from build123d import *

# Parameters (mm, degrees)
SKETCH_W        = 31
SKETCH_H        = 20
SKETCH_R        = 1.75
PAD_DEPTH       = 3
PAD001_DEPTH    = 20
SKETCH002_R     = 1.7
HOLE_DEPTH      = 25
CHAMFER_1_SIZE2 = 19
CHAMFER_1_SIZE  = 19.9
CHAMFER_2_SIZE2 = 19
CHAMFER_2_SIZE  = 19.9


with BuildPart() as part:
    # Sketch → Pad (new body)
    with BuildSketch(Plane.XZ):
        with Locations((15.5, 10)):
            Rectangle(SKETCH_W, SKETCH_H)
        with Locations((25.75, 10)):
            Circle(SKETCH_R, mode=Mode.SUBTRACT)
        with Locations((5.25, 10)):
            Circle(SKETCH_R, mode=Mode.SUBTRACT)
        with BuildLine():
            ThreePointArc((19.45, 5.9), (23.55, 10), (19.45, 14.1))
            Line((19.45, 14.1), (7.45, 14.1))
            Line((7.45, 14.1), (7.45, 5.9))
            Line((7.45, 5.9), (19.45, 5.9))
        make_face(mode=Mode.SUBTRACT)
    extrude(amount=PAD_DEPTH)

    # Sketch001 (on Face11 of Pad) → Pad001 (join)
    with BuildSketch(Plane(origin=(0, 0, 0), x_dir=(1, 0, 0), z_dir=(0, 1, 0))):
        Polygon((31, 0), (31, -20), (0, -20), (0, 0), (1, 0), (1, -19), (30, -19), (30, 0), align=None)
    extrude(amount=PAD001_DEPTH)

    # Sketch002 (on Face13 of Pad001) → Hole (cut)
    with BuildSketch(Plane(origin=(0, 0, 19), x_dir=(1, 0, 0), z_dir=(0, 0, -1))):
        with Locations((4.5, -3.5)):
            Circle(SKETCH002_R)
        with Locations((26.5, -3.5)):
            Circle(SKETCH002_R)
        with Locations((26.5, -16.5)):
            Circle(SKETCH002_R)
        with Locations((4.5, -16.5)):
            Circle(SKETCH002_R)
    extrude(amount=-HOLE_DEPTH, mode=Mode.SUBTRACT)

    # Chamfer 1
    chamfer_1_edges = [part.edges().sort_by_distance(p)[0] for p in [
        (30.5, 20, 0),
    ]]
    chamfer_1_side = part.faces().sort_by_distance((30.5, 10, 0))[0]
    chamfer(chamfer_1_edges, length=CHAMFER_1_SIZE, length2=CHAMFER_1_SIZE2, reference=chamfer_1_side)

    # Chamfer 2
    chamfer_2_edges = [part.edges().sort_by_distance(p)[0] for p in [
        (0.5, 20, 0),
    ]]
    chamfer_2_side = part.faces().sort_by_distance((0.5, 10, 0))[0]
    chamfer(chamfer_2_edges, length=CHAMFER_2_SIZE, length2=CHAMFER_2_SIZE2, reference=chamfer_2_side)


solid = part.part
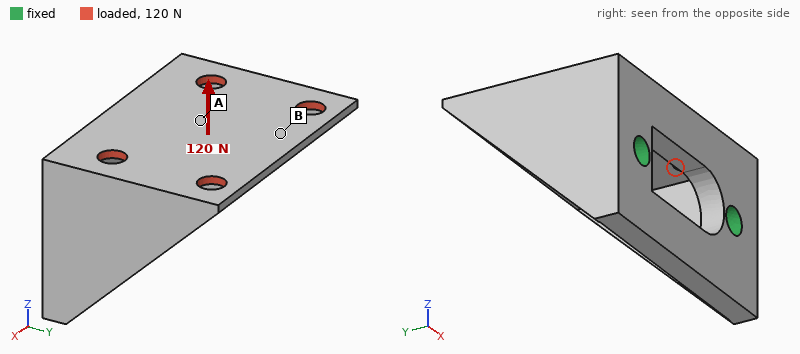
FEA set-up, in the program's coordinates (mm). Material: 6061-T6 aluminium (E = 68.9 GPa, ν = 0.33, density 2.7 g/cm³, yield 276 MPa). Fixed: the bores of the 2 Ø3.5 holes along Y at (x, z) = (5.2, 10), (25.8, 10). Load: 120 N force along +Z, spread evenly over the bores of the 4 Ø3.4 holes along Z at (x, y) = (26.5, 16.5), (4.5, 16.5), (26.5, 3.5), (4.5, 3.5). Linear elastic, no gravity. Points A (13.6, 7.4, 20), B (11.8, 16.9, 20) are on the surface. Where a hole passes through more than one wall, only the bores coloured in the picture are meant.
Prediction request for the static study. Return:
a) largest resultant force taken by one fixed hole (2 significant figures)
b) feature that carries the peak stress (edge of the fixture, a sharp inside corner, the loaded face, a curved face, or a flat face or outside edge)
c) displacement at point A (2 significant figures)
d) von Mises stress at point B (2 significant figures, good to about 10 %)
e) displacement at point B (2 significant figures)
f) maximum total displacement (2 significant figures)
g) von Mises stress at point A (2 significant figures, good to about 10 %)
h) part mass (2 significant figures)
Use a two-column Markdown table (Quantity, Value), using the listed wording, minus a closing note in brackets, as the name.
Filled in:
| Quantity | Value |
|---|---|
| largest resultant force taken by one fixed hole | 65 N |
| feature that carries the peak stress | the loaded face |
| displacement at point A | 0.033 mm |
| von Mises stress at point B | 17 MPa |
| displacement at point B | 0.085 mm |
| maximum total displacement | 0.11 mm |
| von Mises stress at point A | 8.1 MPa |
| part mass | 6.5 g |
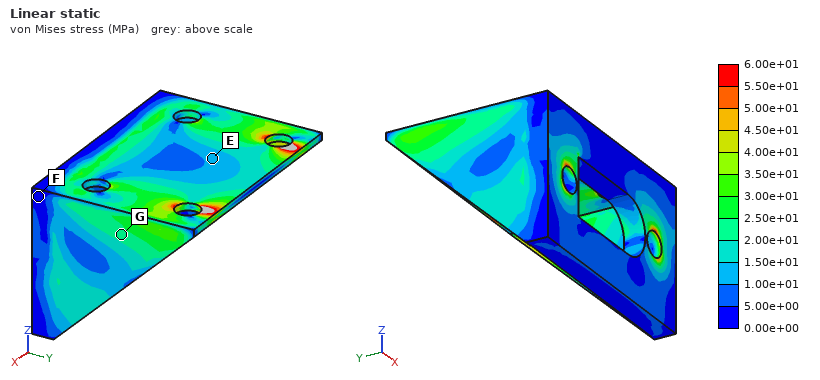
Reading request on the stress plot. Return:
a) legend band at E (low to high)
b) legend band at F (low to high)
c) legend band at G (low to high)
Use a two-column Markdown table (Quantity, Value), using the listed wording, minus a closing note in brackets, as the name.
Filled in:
| Quantity | Value |
|---|---|
| legend band at E | 1.00e+01 to 1.50e+01 MPa |
| legend band at F | 0.00e+00 to 5.00e+00 MPa |
| legend band at G | 2.00e+01 to 2.50e+01 MPa |
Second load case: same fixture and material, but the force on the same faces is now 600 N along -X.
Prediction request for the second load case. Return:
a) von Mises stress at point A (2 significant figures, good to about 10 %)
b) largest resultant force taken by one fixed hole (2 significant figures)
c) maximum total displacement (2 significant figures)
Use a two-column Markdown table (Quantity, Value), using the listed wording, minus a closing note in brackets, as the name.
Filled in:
| Quantity | Value |
|---|---|
| von Mises stress at point A | 15 MPa |
| largest resultant force taken by one fixed hole | 440 N |
| maximum total displacement | 93 µm |
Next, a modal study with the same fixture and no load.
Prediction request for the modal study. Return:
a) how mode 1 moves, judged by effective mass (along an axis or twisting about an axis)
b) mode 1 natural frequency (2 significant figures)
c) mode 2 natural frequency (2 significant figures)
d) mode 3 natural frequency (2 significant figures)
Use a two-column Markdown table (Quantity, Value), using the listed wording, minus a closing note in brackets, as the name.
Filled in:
| Quantity | Value |
|---|---|
| how mode 1 moves, judged by effective mass | along Z |
| mode 1 natural frequency | 4500 Hz |
| mode 2 natural frequency | 8700 Hz |
| mode 3 natural frequency | 11 kHz |
